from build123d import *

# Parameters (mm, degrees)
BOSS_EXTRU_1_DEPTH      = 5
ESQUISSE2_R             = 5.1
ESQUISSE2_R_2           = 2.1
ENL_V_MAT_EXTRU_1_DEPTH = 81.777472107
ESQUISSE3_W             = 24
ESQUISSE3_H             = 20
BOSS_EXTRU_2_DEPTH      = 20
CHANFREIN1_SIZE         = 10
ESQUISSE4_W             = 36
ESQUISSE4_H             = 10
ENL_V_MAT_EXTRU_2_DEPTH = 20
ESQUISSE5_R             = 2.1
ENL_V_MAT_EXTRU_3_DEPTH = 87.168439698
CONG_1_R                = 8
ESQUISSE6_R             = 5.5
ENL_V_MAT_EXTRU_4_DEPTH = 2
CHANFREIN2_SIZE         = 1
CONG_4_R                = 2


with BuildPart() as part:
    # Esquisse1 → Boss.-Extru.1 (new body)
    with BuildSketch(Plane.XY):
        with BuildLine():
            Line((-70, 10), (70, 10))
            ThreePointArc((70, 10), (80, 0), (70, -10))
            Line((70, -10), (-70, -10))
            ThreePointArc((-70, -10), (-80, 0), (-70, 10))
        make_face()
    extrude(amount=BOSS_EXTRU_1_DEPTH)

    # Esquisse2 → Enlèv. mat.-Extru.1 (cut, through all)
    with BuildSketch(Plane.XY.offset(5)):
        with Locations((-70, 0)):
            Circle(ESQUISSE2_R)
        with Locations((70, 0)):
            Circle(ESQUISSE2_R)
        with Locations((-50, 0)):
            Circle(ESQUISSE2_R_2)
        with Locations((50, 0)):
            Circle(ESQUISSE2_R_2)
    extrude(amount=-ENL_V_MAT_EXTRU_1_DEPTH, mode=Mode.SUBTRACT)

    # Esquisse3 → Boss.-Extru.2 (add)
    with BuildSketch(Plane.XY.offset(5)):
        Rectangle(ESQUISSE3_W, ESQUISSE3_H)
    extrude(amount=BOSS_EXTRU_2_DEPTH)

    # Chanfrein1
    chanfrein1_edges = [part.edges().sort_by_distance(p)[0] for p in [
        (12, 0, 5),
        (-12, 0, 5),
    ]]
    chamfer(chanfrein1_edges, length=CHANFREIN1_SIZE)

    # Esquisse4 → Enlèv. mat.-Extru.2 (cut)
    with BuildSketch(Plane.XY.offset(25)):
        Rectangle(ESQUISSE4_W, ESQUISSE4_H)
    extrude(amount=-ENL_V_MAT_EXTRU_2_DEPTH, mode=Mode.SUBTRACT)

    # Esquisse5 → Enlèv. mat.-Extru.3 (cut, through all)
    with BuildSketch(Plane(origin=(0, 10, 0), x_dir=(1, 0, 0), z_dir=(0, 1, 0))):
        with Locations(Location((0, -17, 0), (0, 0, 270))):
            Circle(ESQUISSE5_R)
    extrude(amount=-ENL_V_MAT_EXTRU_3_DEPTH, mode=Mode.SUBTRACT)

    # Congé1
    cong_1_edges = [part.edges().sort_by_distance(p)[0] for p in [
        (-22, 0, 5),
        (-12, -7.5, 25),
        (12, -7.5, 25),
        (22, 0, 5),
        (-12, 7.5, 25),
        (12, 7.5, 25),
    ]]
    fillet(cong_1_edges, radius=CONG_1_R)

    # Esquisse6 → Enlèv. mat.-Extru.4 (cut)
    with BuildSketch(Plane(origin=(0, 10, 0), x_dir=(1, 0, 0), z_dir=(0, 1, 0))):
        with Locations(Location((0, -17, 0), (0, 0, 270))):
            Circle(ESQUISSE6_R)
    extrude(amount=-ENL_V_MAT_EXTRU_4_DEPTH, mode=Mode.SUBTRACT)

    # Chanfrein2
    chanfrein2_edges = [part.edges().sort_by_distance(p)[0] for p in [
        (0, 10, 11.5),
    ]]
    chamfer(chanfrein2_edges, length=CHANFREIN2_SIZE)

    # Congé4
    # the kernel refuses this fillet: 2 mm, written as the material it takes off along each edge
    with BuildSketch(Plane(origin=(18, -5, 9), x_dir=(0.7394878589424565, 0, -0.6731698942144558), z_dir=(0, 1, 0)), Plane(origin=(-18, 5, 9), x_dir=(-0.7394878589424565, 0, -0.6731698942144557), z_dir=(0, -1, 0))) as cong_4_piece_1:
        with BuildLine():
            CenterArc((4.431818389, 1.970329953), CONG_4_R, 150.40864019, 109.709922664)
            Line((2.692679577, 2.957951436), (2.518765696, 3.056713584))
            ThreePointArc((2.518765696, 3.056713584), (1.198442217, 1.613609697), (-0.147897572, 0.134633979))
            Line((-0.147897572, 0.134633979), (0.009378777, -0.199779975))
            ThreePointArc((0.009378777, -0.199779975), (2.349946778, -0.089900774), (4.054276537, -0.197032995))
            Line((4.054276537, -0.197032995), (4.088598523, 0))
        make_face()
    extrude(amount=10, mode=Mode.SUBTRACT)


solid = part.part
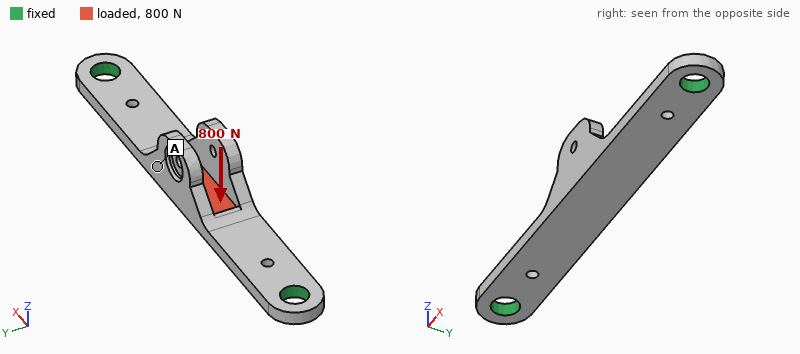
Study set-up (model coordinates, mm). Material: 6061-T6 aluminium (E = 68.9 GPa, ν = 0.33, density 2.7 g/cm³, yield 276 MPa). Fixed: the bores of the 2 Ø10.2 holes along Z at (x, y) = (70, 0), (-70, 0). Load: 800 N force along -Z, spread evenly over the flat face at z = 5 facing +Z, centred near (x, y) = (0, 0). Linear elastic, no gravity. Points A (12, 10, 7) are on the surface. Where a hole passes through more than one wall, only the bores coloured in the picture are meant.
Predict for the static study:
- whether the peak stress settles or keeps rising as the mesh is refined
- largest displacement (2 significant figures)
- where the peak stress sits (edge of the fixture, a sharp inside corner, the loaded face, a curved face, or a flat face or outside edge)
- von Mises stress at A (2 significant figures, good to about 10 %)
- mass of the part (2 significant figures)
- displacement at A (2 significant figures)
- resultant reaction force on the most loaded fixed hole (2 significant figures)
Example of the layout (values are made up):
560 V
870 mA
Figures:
keeps rising
0.28 mm
edge of the fixture
18 MPa
54 g
0.28 mm
570 N
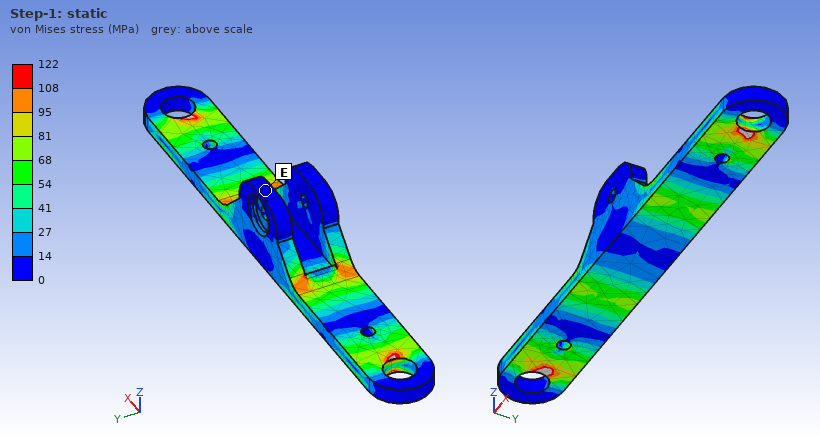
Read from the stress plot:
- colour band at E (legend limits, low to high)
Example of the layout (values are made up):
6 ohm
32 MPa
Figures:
0 to 14 MPa
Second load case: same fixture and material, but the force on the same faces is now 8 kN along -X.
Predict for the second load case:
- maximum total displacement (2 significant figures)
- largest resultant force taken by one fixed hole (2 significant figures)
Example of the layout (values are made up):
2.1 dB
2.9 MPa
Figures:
93 µm
4.0 kN
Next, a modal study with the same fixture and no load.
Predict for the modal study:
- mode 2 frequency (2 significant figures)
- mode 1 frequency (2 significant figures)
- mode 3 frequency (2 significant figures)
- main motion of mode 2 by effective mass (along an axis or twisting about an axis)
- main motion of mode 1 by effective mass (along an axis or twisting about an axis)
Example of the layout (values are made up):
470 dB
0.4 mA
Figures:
2200 Hz
1500 Hz
3700 Hz
along Y
along Z
